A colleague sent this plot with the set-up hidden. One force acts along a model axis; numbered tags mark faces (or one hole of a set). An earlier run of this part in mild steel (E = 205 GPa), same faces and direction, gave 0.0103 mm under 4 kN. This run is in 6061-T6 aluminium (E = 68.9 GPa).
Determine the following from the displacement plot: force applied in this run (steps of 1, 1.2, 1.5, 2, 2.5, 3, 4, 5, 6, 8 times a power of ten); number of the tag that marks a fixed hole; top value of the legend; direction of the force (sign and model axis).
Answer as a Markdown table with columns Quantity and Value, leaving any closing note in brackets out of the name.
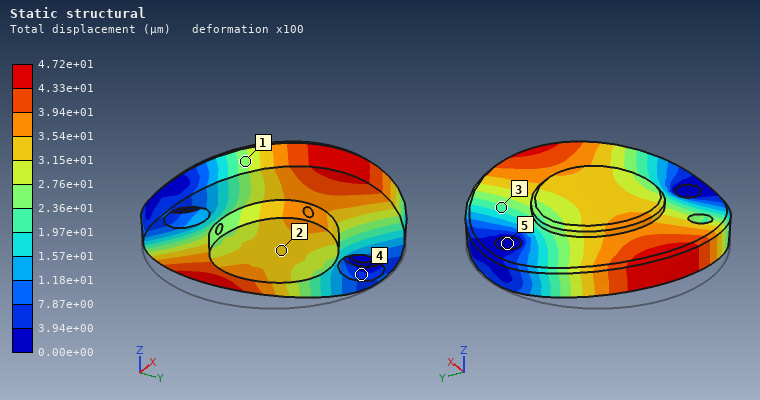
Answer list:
| Quantity | Value |
|---|---|
| force applied in this run | 6 kN |
| number of the tag that marks a fixed hole | 5 |
| top value of the legend | 4.72e+01 µm |
| direction of the force | +Z |
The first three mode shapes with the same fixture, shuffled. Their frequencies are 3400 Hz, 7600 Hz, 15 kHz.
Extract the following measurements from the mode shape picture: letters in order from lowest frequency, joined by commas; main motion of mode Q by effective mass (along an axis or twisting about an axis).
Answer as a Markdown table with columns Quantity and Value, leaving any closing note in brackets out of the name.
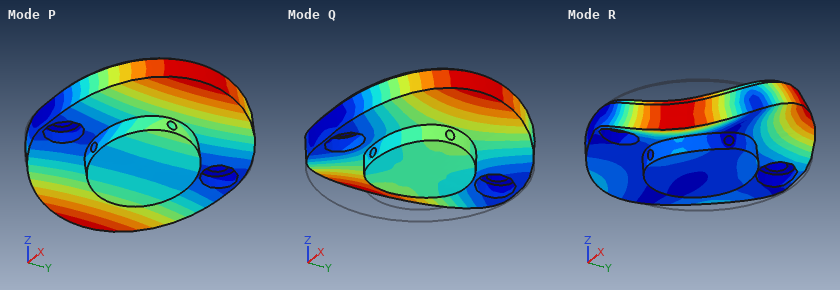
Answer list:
| Quantity | Value |
|---|---|
| letters in order from lowest frequency, joined by commas | P, Q, R |
| main motion of mode Q by effective mass | along Z |
